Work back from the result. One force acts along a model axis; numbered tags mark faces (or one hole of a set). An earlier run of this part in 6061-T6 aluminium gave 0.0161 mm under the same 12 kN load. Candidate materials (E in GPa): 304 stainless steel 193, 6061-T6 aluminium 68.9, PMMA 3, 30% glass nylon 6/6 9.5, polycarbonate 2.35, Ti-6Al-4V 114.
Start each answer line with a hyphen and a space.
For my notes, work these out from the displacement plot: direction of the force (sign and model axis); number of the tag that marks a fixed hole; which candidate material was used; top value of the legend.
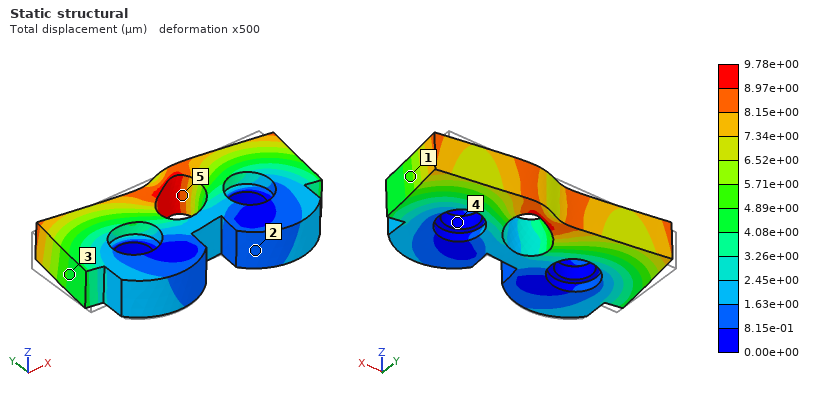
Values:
- +X
- 4
- Ti-6Al-4V
- 9.78e+00 µm
